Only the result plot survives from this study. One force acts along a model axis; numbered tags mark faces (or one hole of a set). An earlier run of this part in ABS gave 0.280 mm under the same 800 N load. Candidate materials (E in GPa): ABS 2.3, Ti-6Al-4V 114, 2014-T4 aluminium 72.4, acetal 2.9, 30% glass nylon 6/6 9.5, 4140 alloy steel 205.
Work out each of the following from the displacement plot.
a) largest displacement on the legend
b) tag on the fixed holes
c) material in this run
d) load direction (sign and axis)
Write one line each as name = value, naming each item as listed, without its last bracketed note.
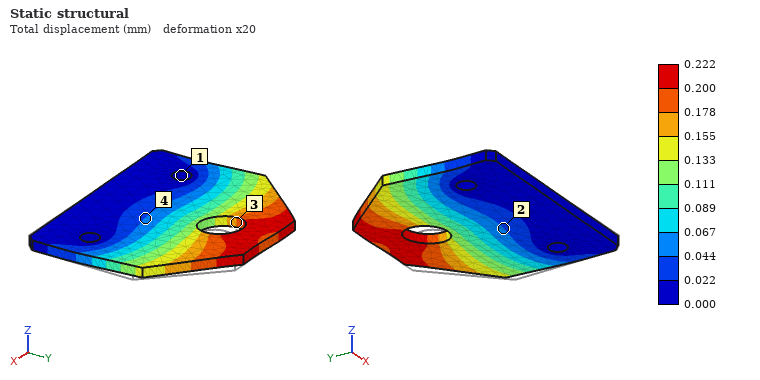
largest displacement on the legend = 0.222 mm
tag on the fixed holes = 1
material in this run = acetal
load direction = -X
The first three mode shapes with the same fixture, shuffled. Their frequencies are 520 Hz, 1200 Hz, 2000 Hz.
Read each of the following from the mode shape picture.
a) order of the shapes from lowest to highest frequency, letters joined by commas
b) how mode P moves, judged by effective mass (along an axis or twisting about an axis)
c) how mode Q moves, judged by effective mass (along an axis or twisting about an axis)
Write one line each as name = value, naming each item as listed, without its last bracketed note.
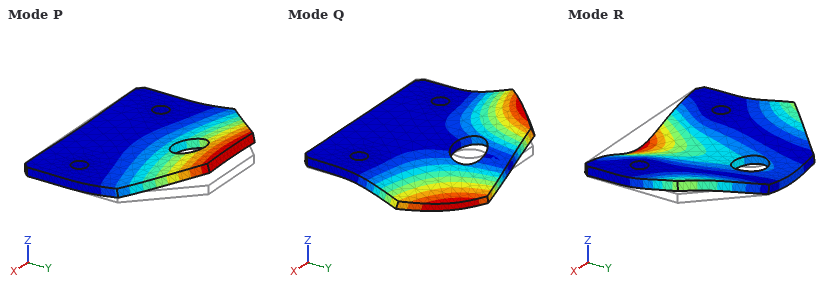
order of the shapes from lowest to highest frequency, letters joined by commas = P, Q, R
how mode P moves, judged by effective mass = along Z
how mode Q moves, judged by effective mass = twisting about Y
